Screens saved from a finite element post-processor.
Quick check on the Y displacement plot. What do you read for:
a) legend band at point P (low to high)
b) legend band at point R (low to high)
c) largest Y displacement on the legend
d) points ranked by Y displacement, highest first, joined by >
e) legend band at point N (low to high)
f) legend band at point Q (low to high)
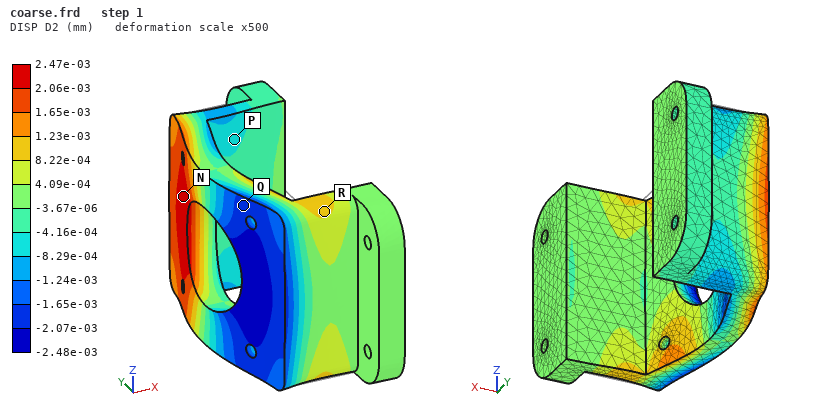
-8.29e-04 to -4.16e-04 mm
8.22e-04 to 1.23e-03 mm
2.47e-03 mm
N > R > P > Q
2.06e-03 to 2.47e-03 mm
-2.07e-03 to -1.65e-03 mm
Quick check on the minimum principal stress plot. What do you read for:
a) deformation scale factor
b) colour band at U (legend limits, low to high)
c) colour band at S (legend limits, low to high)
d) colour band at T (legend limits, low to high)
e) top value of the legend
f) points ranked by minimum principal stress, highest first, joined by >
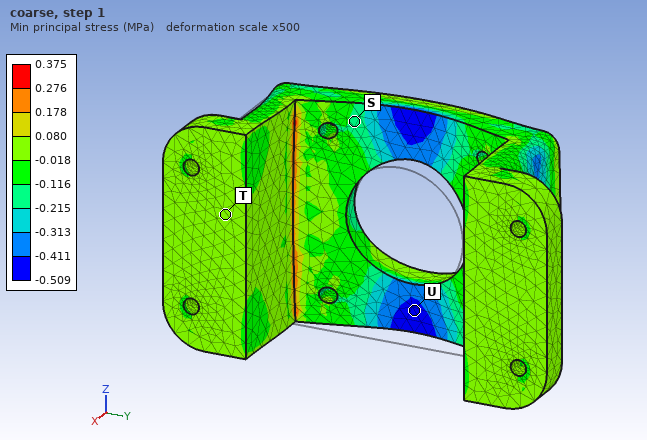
500
-0.509 to -0.411 MPa
-0.215 to -0.116 MPa
-0.018 to 0.080 MPa
0.375 MPa
T > S > U
